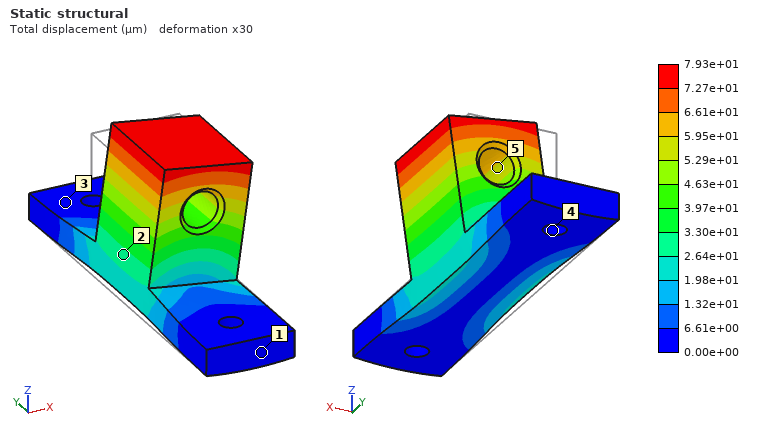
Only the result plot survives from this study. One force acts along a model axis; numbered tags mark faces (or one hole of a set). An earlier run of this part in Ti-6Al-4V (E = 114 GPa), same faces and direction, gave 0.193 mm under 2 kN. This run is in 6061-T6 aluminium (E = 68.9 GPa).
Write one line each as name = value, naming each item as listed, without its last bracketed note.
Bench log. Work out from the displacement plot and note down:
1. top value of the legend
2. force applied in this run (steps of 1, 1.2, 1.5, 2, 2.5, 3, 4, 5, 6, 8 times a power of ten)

top value of the legend = 7.93e+01 µm
force applied in this run = 500 N
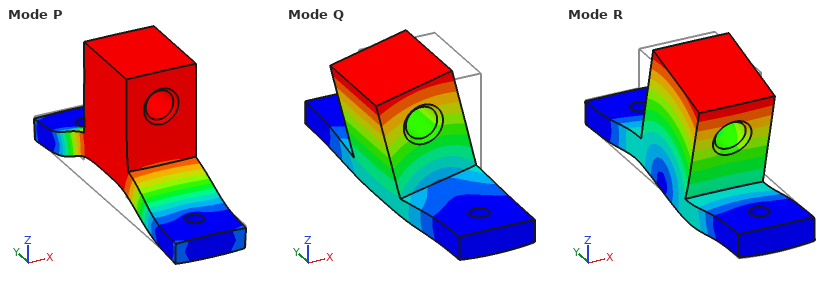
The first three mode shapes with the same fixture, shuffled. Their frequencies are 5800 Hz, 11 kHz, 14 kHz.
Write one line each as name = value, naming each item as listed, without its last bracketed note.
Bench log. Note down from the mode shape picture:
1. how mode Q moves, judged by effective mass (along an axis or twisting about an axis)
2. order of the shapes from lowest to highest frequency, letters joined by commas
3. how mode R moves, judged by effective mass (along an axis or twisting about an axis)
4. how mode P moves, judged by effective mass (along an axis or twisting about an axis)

how mode Q moves, judged by effective mass = along X
order of the shapes from lowest to highest frequency, letters joined by commas = Q, P, R
how mode R moves, judged by effective mass = along Y
how mode P moves, judged by effective mass = along Z
